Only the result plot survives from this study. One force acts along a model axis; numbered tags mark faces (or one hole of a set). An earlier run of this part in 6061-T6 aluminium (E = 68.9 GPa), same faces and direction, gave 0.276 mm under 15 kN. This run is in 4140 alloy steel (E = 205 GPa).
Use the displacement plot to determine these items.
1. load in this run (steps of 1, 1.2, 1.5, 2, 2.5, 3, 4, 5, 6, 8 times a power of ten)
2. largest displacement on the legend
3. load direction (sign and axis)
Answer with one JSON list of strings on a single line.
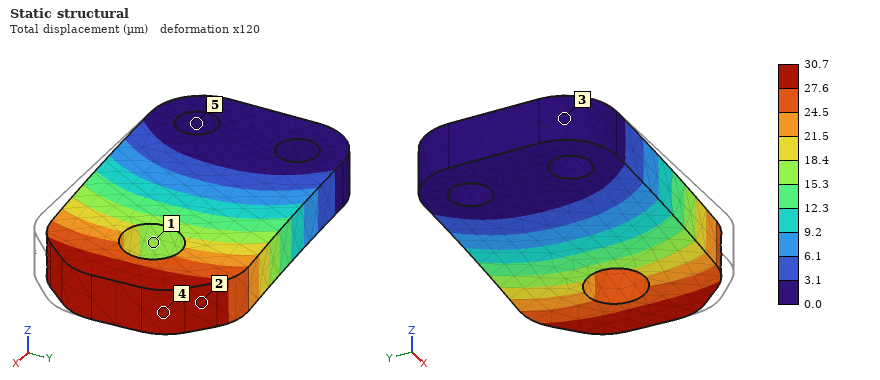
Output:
["5 kN", "30.7 µm", "+Y"]
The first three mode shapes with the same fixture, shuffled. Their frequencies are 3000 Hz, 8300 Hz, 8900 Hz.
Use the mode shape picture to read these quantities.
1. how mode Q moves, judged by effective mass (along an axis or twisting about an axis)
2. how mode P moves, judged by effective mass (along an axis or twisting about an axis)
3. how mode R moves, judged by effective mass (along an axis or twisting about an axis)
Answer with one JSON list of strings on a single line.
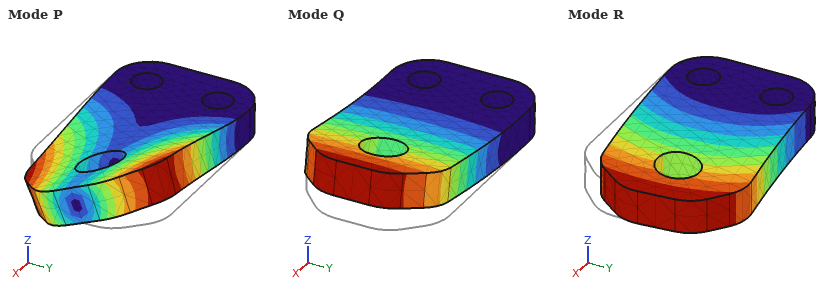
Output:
["along Z", "twisting about X", "along Y"]
